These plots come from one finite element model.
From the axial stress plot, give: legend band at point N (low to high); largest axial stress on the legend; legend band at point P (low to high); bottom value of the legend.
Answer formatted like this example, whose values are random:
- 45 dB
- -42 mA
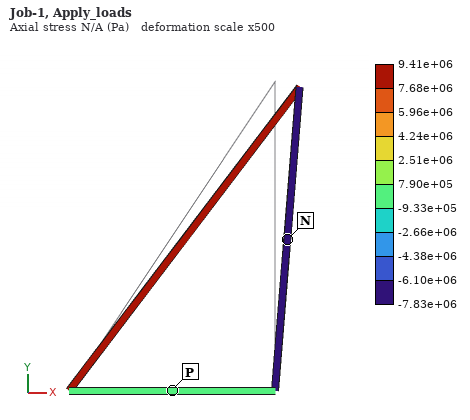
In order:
- -7.83e+06 to -6.10e+06 Pa
- 9.41e+06 Pa
- -9.33e+05 to 7.90e+05 Pa
- -7.83e+06 Pa
